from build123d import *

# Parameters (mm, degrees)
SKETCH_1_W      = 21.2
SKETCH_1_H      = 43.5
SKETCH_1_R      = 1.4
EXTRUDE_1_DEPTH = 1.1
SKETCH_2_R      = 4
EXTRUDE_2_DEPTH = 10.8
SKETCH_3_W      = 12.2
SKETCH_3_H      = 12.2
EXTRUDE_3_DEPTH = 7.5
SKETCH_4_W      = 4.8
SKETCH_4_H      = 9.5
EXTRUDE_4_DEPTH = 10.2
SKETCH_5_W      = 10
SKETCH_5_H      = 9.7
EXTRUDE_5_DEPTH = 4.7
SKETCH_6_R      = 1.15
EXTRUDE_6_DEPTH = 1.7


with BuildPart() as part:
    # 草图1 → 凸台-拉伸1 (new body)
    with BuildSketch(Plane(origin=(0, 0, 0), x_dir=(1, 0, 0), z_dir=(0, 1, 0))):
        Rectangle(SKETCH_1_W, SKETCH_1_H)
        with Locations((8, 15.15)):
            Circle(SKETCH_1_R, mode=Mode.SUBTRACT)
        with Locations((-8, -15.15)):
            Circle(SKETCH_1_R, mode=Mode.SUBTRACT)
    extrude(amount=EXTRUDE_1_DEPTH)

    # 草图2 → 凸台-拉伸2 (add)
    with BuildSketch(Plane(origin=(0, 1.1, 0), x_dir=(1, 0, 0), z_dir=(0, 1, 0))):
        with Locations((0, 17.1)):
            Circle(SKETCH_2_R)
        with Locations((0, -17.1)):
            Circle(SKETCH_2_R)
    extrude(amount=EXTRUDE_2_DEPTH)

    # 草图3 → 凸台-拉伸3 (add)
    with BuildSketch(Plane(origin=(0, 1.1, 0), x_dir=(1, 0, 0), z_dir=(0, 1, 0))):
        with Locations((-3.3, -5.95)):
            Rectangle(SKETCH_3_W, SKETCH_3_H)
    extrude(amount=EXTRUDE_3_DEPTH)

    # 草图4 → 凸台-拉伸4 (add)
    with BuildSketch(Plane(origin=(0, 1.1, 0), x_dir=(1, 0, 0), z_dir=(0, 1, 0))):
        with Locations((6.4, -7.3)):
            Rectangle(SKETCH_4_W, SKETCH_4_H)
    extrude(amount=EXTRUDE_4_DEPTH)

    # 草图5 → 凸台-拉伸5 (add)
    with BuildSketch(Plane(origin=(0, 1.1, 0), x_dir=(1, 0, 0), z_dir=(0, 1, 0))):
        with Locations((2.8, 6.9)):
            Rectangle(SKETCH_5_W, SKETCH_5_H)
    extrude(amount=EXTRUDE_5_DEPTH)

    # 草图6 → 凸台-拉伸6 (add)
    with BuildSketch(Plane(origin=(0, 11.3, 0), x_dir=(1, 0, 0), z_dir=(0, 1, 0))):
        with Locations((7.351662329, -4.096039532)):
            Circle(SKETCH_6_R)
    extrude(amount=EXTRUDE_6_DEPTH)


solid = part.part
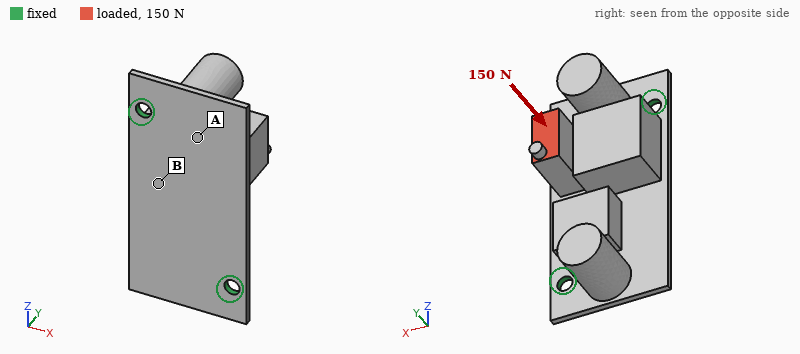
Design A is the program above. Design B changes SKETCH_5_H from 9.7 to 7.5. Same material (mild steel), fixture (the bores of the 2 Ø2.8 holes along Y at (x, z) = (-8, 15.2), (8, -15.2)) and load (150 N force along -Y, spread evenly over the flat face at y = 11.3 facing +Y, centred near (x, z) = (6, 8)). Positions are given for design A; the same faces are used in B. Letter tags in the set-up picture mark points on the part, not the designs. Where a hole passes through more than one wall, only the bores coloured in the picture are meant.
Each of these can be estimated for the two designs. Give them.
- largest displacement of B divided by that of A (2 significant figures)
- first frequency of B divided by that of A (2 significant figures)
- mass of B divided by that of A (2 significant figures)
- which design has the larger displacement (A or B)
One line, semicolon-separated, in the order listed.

1.1; 0.97; 0.97; B
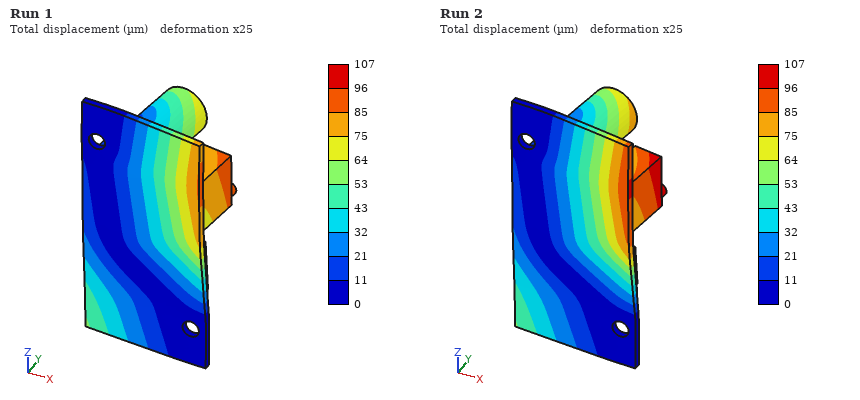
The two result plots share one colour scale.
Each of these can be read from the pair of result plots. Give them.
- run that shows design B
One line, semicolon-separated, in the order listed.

Run 2
